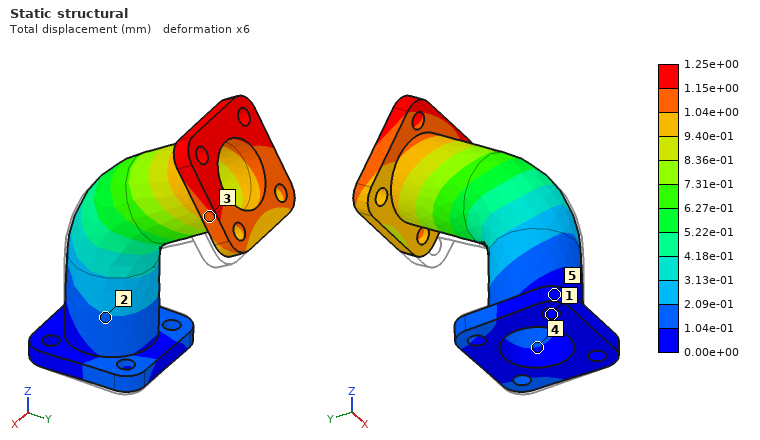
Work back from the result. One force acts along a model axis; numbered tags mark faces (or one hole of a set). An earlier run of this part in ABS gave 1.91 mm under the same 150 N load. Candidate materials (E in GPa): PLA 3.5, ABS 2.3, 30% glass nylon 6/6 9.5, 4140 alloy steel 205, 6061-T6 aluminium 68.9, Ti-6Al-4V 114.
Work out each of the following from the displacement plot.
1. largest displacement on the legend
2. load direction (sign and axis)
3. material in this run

1.25e+00 mm
-X
PLA
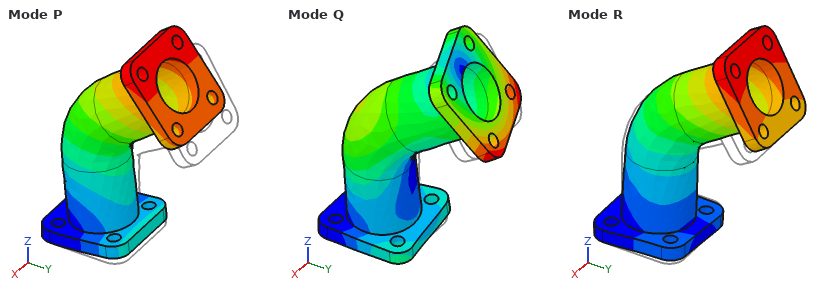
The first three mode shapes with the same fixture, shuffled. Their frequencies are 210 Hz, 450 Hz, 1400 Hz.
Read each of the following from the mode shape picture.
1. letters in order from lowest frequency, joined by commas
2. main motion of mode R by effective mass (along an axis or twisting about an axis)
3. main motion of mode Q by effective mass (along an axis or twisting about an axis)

P, R, Q
along X
twisting about Z
